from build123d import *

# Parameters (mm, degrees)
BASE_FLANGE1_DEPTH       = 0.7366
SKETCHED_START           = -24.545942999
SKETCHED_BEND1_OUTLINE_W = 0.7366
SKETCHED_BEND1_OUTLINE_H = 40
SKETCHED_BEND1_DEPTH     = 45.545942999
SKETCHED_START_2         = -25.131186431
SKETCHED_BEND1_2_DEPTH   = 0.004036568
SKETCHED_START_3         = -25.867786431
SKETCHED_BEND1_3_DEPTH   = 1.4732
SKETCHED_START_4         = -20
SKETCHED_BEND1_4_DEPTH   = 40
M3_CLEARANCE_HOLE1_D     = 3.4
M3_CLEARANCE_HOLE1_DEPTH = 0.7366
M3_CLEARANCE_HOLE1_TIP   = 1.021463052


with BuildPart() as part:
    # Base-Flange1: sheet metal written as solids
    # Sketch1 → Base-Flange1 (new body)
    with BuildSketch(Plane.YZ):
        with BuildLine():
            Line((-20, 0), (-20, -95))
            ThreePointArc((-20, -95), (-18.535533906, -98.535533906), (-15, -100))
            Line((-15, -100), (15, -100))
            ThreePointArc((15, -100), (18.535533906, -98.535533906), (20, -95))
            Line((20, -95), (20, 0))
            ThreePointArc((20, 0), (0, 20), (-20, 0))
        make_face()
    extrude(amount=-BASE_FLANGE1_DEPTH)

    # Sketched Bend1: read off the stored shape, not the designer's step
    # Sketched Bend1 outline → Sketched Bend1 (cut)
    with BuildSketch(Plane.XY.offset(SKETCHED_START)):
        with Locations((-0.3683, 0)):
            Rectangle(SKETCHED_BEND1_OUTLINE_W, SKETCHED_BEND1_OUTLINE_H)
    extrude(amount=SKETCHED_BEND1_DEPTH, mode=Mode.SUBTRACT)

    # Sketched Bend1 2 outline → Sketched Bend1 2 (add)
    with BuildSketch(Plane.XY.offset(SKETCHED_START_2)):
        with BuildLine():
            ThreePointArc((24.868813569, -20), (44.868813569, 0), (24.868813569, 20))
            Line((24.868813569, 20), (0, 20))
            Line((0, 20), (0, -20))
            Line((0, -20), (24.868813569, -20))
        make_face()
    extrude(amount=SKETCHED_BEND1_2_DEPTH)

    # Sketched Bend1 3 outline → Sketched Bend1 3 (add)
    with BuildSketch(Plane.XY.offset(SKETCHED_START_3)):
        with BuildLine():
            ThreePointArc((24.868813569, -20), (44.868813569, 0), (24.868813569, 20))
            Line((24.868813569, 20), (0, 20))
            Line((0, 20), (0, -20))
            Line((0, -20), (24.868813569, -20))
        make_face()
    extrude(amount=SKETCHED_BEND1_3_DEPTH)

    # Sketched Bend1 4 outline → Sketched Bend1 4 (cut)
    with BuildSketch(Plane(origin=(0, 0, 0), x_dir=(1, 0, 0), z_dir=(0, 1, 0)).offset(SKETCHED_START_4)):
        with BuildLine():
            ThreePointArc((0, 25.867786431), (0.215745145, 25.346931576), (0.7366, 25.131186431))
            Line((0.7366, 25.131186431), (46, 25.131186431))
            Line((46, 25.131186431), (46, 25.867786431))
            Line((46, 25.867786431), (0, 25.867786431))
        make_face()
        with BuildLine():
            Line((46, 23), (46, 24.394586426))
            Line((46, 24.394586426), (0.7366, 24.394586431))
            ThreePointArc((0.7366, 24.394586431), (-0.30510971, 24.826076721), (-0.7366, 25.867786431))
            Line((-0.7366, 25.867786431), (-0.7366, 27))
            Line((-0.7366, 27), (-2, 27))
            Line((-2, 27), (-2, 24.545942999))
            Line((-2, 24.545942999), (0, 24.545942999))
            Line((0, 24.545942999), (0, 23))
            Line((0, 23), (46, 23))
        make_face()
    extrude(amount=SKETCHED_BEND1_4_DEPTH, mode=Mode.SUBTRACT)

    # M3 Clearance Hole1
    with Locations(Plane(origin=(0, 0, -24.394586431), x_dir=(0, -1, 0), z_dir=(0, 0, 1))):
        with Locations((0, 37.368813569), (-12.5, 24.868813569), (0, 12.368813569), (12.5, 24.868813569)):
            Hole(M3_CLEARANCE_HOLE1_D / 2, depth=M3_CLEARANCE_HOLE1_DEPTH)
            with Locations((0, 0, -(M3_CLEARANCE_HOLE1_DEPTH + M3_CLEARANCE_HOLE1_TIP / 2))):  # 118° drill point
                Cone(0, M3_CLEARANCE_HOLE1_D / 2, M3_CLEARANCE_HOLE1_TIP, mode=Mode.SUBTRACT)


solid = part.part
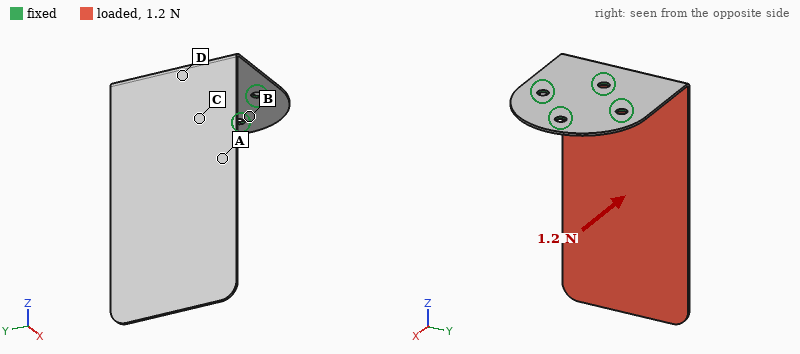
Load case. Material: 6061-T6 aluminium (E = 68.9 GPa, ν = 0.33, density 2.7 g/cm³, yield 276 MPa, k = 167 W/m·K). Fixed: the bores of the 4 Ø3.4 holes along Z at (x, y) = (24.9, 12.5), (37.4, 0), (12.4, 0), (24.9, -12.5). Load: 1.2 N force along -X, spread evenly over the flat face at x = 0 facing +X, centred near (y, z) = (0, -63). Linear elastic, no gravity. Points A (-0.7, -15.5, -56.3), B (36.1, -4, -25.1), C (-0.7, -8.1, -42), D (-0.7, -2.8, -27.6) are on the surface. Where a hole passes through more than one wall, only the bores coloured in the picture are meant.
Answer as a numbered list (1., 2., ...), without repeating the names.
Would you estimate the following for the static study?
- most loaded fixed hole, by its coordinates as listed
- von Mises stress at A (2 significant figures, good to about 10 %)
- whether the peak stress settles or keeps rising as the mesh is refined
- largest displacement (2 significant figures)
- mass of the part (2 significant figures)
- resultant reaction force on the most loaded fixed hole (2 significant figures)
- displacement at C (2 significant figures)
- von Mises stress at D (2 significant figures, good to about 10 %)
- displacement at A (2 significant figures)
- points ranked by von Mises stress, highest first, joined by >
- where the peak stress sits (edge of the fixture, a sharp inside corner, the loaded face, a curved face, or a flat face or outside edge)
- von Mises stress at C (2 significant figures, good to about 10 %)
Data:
1. (12.4, 0)
2. 4.3 MPa
3. keeps rising
4. 1.1 mm
5. 9.1 g
6. 2.0 N
7. 0.17 mm
8. 10 MPa
9. 0.36 mm
10. D > C > A > B
11. edge of the fixture
12. 6.8 MPa
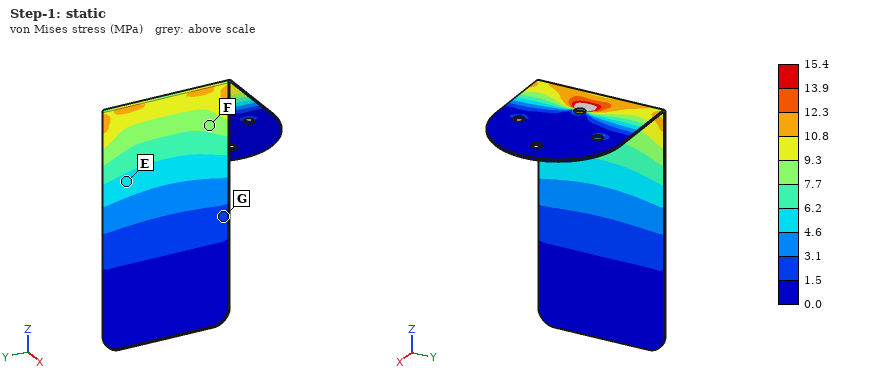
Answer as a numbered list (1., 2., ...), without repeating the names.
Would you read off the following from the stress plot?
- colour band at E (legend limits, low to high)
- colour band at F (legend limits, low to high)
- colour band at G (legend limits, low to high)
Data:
1. 4.6 to 6.2 MPa
2. 7.7 to 9.3 MPa
3. 1.5 to 3.1 MPa
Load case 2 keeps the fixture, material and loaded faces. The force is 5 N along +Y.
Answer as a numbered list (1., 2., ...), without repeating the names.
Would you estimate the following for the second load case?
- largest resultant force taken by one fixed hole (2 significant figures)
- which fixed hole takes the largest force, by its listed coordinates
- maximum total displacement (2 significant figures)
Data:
1. 4.7 N
2. (12.4, 0)
3. 0.98 mm
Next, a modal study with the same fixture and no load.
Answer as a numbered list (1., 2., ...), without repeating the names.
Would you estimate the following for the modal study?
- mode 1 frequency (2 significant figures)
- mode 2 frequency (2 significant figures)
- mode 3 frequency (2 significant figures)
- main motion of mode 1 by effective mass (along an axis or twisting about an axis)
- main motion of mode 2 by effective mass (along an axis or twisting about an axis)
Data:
1. 85 Hz
2. 180 Hz
3. 430 Hz
4. along X
5. along Y
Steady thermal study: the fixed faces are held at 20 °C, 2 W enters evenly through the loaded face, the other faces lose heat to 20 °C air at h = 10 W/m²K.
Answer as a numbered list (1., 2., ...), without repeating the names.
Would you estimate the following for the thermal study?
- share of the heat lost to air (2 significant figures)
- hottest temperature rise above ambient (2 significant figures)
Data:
1. 23 %
2. 17 K
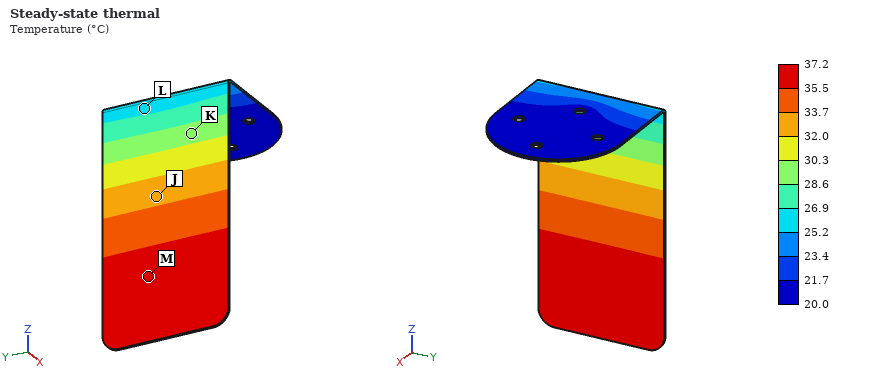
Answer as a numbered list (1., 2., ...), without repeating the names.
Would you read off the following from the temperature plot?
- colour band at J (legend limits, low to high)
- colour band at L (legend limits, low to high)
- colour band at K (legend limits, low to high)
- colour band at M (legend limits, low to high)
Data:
1. 32.0 to 33.7 °C
2. 25.2 to 26.9 °C
3. 28.6 to 30.3 °C
4. 35.5 to 37.2 °C
